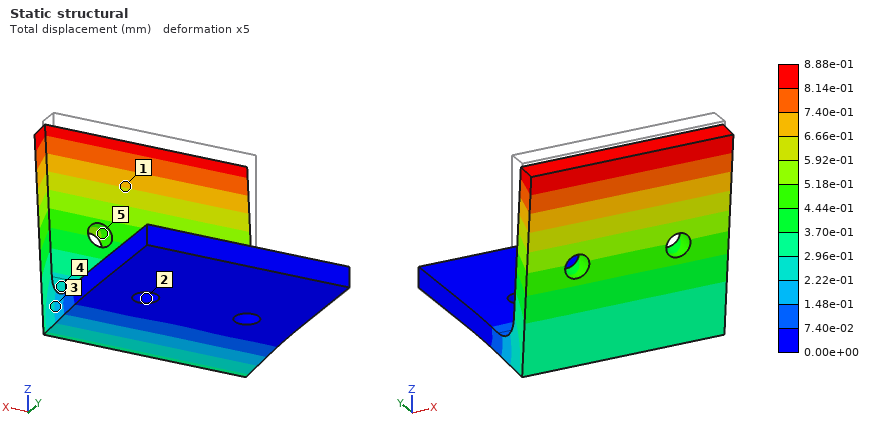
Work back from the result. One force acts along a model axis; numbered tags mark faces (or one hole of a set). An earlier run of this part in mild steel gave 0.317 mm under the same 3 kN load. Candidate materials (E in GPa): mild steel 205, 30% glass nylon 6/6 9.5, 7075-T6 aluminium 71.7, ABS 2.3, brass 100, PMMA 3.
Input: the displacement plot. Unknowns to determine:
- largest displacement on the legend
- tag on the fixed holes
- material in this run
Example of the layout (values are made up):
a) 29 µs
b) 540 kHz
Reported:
a) 8.88e-01 mm
b) 2
c) 7075-T6 aluminium
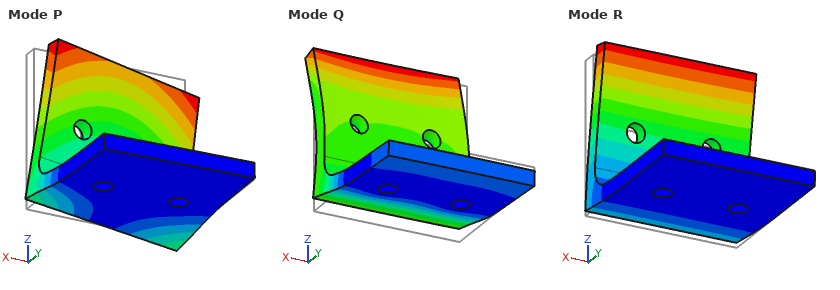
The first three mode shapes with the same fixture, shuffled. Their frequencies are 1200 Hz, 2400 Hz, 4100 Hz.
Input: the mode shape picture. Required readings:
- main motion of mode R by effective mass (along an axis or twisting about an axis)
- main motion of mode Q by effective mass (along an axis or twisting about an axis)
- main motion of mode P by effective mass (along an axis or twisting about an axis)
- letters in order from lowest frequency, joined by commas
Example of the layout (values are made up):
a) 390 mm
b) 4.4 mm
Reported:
a) along Y
b) along Z
c) along X
d) R, P, Q
